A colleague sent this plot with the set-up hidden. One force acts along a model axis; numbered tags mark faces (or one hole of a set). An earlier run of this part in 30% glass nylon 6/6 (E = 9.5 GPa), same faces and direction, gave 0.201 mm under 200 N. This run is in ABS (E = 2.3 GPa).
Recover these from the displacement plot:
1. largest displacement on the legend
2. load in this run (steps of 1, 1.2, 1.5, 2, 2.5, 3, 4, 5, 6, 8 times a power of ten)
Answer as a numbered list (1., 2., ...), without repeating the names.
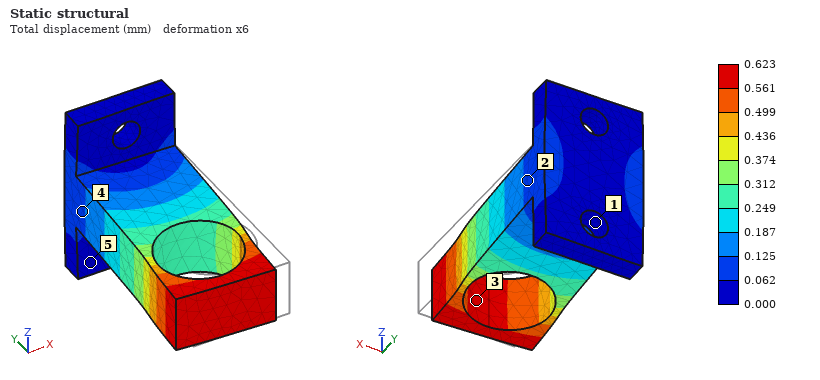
1. 0.623 mm
2. 150 N
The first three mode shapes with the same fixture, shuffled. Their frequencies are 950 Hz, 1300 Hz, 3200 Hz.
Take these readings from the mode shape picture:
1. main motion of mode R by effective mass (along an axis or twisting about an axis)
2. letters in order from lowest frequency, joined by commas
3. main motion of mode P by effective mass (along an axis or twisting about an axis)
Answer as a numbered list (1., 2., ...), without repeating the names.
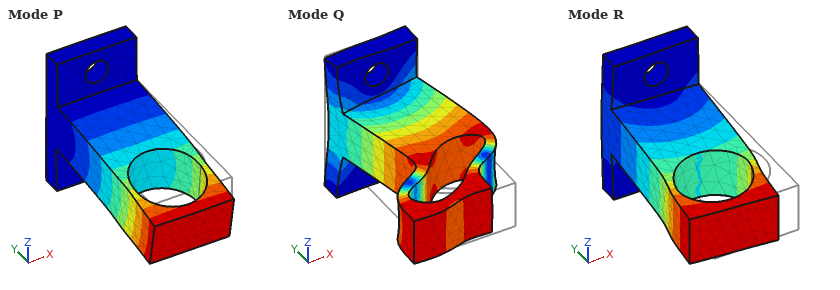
1. along X
2. R, P, Q
3. along Z
